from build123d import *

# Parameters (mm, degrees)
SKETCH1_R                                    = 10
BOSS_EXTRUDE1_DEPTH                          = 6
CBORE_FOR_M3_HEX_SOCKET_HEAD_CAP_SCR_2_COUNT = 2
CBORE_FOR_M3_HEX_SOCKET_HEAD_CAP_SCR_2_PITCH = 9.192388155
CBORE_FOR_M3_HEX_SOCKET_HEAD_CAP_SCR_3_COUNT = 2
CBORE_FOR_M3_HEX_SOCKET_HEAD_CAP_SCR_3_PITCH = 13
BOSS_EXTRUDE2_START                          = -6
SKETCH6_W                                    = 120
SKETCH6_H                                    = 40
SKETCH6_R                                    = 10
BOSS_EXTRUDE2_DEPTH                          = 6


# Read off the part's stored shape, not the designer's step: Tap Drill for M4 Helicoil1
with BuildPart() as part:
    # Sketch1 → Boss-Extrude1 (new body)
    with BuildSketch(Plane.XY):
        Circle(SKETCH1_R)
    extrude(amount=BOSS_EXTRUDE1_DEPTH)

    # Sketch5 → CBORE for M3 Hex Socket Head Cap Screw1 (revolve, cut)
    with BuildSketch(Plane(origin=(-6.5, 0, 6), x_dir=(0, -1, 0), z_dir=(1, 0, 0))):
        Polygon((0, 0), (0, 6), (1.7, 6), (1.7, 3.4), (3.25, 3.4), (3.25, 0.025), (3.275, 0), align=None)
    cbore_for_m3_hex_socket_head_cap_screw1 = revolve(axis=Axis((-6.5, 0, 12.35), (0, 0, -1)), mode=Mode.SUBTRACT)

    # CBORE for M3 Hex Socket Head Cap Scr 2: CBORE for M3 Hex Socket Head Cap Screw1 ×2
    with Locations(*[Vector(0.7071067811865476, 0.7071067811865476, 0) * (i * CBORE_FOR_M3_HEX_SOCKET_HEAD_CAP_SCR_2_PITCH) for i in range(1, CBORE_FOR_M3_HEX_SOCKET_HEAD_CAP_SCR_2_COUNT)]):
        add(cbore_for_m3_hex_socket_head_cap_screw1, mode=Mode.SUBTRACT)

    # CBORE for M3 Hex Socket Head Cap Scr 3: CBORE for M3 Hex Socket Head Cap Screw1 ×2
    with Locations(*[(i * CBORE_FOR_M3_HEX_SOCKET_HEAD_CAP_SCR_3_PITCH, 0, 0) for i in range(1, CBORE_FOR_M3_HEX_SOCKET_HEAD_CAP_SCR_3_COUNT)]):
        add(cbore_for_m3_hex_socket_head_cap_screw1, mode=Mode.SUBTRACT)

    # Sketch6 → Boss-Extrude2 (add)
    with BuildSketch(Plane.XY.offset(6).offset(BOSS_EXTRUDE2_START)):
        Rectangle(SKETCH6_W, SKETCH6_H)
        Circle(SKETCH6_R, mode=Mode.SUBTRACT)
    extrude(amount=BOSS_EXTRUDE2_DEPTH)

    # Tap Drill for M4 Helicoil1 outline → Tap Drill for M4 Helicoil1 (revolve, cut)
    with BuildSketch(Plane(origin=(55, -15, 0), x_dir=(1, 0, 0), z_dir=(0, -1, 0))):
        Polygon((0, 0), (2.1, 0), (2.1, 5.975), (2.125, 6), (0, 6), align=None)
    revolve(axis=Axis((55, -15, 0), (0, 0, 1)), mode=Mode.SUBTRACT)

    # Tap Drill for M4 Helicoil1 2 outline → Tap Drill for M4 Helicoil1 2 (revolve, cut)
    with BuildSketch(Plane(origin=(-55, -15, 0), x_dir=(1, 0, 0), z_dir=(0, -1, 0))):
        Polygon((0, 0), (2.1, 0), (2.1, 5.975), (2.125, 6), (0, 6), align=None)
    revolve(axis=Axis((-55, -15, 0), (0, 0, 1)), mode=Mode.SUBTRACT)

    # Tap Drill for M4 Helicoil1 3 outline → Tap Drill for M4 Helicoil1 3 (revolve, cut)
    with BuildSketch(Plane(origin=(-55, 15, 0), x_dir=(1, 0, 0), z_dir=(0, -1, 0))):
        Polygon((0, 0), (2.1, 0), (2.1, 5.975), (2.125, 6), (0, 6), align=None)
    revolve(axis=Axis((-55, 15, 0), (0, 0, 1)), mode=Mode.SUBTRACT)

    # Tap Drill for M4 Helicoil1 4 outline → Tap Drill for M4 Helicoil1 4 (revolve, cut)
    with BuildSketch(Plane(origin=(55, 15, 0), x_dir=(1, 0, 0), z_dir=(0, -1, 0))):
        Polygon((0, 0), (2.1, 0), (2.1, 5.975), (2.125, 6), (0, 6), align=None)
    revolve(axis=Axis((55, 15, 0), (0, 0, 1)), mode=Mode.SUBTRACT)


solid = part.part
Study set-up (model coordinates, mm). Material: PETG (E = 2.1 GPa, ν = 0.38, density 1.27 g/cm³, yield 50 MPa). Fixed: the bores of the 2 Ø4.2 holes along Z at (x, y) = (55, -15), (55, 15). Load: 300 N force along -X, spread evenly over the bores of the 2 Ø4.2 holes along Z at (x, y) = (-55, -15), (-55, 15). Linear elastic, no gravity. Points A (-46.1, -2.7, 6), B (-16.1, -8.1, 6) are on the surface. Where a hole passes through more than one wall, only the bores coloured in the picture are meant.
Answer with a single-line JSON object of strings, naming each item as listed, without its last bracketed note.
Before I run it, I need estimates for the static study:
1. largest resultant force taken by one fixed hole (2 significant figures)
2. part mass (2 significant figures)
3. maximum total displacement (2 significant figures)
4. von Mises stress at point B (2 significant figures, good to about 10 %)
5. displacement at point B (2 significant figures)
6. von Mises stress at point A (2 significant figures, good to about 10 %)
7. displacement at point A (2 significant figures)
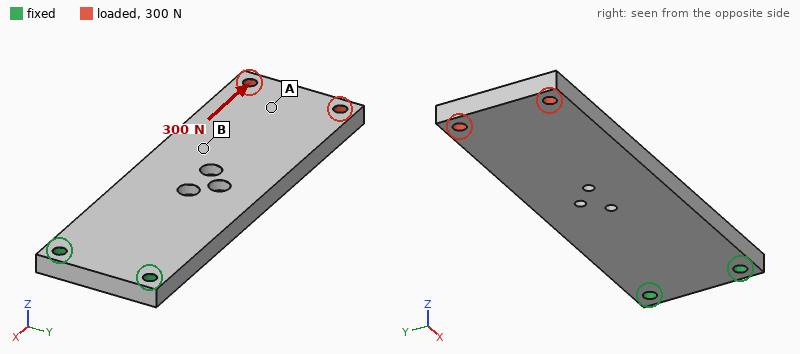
{"largest resultant force taken by one fixed hole": "150 N", "part mass": "36 g", "maximum total displacement": "93 µm", "von Mises stress at point B": "1.4 MPa", "displacement at point B": "51 µm", "von Mises stress at point A": "0.58 MPa", "displacement at point A": "69 µm"}
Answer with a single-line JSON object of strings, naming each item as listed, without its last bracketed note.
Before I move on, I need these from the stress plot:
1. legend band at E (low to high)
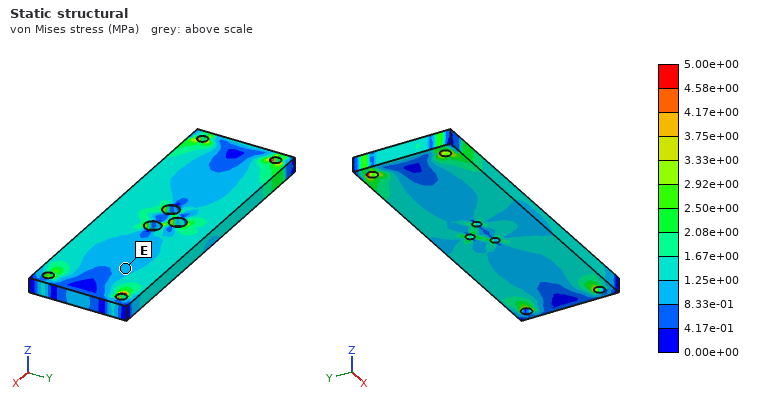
{"legend band at E": "8.33e-01 to 1.25e+00 MPa"}
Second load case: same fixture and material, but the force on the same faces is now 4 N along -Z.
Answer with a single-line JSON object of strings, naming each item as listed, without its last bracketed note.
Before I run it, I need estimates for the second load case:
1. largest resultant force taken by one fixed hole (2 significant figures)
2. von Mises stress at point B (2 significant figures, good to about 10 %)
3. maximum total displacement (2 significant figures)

{"largest resultant force taken by one fixed hole": "2.0 N", "von Mises stress at point B": "0.68 MPa", "maximum total displacement": "1.3 mm"}
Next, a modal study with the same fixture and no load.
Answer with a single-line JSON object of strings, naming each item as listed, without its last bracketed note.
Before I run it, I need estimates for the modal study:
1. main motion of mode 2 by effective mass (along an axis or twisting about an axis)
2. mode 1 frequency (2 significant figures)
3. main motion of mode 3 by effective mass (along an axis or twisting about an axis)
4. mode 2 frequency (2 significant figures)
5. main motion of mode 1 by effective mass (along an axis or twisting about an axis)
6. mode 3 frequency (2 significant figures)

{"main motion of mode 2 by effective mass": "twisting about X", "mode 1 frequency": "92 Hz", "main motion of mode 3 by effective mass": "along Z", "mode 2 frequency": "520 Hz", "main motion of mode 1 by effective mass": "along Z", "mode 3 frequency": "570 Hz"}
